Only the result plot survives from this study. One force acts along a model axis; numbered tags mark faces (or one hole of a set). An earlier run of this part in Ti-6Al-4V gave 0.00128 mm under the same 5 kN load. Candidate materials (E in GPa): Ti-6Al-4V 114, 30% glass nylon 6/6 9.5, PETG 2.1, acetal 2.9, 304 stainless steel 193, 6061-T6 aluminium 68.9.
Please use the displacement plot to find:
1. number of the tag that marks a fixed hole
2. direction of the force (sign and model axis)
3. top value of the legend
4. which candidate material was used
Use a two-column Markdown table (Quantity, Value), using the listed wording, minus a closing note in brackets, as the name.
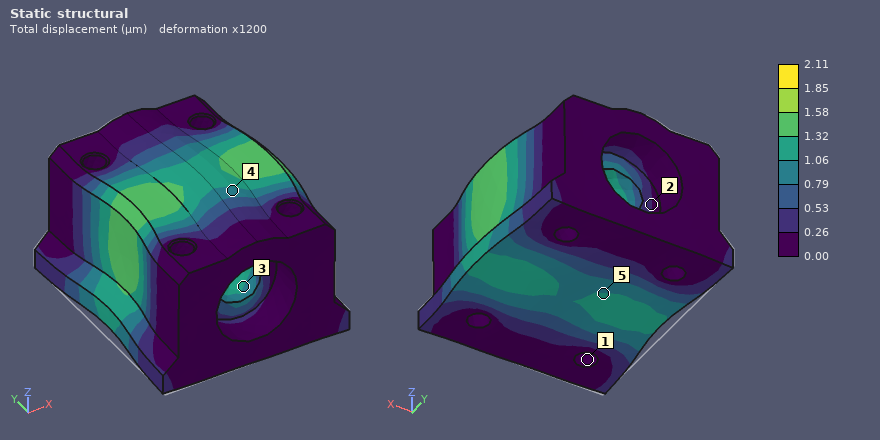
| Quantity | Value |
|---|---|
| number of the tag that marks a fixed hole | 1 |
| direction of the force | +X |
| top value of the legend | 2.11 µm |
| which candidate material was used | 6061-T6 aluminium |
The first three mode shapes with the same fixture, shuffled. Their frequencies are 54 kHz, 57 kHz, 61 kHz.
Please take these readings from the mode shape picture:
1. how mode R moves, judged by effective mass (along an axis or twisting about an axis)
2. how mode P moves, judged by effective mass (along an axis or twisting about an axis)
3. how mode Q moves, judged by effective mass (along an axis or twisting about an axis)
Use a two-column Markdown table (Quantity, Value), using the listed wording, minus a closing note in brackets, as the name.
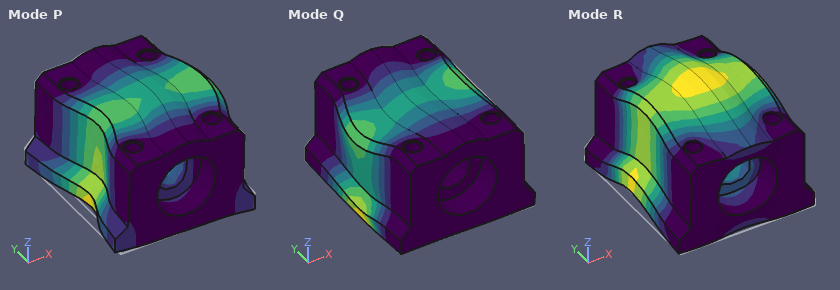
| Quantity | Value |
|---|---|
| how mode R moves, judged by effective mass | along Z |
| how mode P moves, judged by effective mass | along X |
| how mode Q moves, judged by effective mass | twisting about Y |
